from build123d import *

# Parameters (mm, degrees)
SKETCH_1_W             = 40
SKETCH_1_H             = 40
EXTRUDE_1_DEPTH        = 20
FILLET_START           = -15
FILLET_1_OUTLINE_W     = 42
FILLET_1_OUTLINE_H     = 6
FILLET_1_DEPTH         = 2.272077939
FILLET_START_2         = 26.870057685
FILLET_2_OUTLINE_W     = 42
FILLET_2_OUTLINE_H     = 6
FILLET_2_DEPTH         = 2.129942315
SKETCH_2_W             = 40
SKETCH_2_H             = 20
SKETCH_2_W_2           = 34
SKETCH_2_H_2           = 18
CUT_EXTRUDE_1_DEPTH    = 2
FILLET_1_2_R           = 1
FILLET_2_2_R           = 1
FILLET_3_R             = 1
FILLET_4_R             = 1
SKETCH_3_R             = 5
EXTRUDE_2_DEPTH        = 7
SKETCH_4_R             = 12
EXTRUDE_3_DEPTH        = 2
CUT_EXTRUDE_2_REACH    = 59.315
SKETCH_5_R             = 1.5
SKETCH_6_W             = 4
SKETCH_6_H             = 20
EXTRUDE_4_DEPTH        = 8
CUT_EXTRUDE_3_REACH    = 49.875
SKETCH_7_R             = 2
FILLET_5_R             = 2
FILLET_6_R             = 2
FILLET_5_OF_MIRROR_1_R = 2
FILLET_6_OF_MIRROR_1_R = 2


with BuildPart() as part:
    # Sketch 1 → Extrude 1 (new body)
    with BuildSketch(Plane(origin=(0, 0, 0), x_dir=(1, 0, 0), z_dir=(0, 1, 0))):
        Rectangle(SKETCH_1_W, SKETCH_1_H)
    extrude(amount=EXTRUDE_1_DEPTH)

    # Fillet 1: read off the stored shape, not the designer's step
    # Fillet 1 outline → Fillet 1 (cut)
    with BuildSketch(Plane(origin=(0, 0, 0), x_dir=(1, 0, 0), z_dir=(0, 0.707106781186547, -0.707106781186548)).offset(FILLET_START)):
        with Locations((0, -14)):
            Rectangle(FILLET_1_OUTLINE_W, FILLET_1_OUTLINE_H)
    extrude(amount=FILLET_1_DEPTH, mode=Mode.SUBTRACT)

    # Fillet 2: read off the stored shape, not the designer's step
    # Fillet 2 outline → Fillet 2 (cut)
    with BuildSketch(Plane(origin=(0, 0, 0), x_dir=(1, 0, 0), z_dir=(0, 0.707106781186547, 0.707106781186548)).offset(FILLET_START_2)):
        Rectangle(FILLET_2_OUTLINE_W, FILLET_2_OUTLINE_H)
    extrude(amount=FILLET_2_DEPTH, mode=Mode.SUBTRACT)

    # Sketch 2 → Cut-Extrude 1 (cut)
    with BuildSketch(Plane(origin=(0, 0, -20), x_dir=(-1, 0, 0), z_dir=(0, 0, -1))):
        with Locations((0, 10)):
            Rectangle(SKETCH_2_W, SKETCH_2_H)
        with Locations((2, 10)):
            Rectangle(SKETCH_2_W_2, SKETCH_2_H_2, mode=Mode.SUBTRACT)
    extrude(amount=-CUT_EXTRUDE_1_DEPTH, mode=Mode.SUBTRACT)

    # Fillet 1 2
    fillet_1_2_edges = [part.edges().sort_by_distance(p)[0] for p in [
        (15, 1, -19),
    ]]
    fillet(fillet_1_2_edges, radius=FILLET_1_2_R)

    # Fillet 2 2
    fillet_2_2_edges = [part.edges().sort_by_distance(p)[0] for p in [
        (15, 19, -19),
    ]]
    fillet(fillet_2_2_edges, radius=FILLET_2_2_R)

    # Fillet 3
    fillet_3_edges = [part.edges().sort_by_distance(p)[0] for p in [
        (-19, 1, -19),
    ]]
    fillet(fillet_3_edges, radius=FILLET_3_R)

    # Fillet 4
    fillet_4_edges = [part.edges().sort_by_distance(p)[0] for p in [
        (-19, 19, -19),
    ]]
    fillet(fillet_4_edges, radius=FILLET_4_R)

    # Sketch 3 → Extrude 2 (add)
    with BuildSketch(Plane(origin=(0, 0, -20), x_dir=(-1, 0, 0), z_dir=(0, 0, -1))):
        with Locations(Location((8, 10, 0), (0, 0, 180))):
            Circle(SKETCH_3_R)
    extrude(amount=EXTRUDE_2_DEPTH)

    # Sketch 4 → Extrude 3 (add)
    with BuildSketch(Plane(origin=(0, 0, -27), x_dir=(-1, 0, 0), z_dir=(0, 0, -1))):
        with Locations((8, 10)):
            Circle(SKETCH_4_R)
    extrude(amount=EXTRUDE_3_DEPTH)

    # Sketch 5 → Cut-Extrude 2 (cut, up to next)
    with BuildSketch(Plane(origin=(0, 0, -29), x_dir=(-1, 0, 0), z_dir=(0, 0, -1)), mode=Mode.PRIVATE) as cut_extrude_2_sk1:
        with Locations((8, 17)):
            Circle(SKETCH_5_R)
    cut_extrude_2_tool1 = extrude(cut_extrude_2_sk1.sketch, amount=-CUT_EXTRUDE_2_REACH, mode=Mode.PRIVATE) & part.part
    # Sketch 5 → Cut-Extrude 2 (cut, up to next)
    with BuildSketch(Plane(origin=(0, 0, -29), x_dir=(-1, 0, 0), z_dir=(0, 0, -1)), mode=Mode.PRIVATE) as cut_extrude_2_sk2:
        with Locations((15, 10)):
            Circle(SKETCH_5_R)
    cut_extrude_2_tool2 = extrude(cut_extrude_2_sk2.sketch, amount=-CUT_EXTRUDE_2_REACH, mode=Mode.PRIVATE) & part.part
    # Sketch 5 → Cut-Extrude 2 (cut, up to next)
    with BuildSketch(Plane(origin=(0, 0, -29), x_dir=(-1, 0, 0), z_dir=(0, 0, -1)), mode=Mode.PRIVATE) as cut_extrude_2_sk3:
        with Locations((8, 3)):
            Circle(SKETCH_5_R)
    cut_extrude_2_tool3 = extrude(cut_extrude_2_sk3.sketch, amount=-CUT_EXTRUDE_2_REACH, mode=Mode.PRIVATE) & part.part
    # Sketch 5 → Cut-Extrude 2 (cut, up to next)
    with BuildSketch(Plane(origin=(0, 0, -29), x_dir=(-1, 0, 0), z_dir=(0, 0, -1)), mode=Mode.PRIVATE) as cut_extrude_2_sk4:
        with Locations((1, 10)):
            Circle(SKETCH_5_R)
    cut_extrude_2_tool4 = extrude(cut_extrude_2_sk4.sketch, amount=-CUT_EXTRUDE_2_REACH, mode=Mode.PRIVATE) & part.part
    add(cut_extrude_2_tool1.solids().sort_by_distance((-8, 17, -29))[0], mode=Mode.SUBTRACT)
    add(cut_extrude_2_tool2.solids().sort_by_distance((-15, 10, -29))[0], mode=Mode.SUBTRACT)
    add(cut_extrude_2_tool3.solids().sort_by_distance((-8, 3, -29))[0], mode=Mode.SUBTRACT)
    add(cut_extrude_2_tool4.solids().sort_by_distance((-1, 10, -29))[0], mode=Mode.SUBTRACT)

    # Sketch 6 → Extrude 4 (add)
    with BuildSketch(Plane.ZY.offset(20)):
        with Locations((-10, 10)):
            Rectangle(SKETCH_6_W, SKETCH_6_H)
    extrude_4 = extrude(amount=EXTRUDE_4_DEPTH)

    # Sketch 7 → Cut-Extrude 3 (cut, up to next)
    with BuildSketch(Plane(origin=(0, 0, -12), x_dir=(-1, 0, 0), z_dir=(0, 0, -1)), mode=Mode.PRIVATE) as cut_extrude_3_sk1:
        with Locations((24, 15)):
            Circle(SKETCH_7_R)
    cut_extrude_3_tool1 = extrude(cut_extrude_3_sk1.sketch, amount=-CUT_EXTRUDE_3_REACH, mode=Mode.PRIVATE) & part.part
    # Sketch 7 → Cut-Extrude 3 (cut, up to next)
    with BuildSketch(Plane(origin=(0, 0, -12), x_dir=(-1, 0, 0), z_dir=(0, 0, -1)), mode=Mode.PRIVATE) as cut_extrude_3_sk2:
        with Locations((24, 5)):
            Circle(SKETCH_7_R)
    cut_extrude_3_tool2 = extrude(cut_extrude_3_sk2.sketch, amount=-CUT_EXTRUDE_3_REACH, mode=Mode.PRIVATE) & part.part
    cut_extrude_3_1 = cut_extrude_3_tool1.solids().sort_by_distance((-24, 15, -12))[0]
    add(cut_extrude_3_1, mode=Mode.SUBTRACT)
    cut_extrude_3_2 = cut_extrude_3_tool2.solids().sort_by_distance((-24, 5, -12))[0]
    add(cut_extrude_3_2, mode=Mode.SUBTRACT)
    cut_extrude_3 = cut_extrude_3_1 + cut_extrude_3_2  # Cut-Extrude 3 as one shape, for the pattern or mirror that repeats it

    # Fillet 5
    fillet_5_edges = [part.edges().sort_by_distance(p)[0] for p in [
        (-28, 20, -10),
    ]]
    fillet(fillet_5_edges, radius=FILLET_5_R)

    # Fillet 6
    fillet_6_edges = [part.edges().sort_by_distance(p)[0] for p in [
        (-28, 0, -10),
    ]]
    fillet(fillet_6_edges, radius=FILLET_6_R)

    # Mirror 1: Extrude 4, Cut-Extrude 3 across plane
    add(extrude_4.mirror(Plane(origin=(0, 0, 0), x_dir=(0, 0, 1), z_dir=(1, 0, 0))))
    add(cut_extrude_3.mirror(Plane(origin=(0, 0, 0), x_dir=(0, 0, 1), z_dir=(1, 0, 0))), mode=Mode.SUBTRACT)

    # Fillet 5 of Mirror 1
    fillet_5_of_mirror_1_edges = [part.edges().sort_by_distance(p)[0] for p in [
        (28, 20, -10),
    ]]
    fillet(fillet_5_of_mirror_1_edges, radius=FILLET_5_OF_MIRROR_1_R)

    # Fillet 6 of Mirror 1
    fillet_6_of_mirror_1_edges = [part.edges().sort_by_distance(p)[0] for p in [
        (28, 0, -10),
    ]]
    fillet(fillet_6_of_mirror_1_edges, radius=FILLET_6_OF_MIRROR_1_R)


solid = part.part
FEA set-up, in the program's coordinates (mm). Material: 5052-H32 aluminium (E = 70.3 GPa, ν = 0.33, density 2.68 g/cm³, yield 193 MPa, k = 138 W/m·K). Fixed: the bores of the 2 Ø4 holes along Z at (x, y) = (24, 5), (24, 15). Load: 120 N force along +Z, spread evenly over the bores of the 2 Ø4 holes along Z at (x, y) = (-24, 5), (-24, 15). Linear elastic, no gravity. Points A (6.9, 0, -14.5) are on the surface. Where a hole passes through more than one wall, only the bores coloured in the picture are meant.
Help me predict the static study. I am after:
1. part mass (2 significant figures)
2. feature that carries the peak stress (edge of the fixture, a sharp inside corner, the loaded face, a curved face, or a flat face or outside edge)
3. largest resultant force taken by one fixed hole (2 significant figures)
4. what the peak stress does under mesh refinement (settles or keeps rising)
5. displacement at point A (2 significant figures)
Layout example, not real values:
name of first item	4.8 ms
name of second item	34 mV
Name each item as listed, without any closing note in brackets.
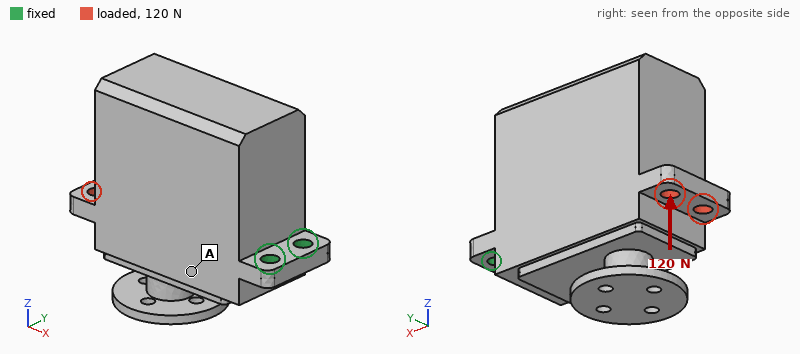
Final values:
part mass	91 g
feature that carries the peak stress	edge of the fixture
largest resultant force taken by one fixed hole	60 N
what the peak stress does under mesh refinement	keeps rising
displacement at point A	0.045 mm
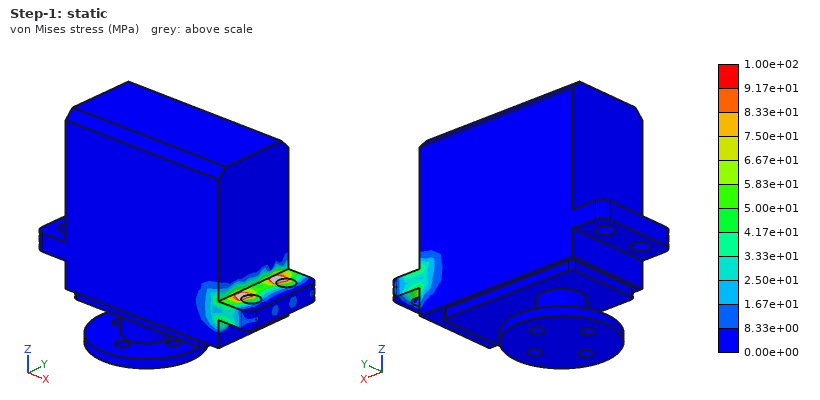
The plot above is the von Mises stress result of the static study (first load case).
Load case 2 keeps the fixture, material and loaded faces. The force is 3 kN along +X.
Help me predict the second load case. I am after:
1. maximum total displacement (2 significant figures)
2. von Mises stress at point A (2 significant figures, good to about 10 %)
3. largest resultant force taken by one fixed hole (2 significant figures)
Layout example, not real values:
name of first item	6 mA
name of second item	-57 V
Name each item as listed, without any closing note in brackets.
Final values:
maximum total displacement	16 µm
von Mises stress at point A	9.2 MPa
largest resultant force taken by one fixed hole	1.5 kN
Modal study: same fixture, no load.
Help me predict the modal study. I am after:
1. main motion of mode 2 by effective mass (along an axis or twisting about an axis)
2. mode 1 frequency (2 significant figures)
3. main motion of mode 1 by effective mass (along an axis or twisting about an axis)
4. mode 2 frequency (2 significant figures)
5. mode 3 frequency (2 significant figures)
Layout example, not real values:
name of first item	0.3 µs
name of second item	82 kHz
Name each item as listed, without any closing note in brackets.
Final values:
main motion of mode 2 by effective mass	along Y
mode 1 frequency	770 Hz
main motion of mode 1 by effective mass	along Z
mode 2 frequency	2600 Hz
mode 3 frequency	4100 Hz
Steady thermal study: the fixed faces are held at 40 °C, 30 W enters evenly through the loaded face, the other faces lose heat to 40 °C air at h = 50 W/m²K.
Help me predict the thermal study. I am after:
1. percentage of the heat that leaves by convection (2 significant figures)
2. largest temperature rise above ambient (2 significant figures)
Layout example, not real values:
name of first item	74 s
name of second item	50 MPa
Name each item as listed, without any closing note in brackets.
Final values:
percentage of the heat that leaves by convection	23 %
largest temperature rise above ambient	46 K
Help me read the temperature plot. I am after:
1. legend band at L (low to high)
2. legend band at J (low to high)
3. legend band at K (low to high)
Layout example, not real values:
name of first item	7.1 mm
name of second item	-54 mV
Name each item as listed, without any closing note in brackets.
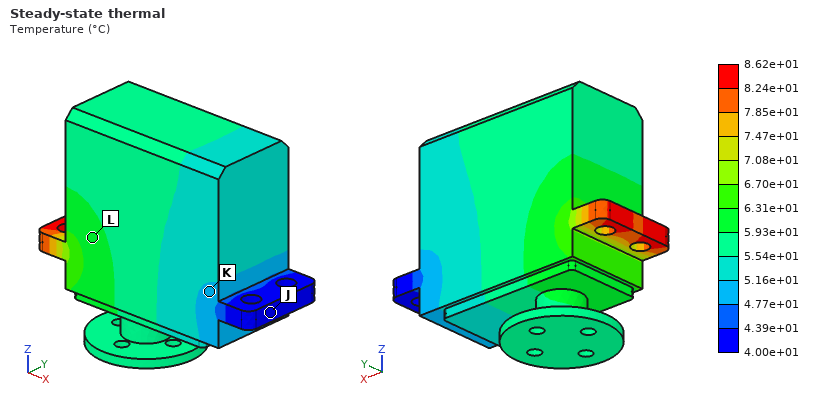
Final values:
legend band at L	5.93e+01 to 6.31e+01 °C
legend band at J	4.00e+01 to 4.39e+01 °C
legend band at K	4.77e+01 to 5.16e+01 °C
